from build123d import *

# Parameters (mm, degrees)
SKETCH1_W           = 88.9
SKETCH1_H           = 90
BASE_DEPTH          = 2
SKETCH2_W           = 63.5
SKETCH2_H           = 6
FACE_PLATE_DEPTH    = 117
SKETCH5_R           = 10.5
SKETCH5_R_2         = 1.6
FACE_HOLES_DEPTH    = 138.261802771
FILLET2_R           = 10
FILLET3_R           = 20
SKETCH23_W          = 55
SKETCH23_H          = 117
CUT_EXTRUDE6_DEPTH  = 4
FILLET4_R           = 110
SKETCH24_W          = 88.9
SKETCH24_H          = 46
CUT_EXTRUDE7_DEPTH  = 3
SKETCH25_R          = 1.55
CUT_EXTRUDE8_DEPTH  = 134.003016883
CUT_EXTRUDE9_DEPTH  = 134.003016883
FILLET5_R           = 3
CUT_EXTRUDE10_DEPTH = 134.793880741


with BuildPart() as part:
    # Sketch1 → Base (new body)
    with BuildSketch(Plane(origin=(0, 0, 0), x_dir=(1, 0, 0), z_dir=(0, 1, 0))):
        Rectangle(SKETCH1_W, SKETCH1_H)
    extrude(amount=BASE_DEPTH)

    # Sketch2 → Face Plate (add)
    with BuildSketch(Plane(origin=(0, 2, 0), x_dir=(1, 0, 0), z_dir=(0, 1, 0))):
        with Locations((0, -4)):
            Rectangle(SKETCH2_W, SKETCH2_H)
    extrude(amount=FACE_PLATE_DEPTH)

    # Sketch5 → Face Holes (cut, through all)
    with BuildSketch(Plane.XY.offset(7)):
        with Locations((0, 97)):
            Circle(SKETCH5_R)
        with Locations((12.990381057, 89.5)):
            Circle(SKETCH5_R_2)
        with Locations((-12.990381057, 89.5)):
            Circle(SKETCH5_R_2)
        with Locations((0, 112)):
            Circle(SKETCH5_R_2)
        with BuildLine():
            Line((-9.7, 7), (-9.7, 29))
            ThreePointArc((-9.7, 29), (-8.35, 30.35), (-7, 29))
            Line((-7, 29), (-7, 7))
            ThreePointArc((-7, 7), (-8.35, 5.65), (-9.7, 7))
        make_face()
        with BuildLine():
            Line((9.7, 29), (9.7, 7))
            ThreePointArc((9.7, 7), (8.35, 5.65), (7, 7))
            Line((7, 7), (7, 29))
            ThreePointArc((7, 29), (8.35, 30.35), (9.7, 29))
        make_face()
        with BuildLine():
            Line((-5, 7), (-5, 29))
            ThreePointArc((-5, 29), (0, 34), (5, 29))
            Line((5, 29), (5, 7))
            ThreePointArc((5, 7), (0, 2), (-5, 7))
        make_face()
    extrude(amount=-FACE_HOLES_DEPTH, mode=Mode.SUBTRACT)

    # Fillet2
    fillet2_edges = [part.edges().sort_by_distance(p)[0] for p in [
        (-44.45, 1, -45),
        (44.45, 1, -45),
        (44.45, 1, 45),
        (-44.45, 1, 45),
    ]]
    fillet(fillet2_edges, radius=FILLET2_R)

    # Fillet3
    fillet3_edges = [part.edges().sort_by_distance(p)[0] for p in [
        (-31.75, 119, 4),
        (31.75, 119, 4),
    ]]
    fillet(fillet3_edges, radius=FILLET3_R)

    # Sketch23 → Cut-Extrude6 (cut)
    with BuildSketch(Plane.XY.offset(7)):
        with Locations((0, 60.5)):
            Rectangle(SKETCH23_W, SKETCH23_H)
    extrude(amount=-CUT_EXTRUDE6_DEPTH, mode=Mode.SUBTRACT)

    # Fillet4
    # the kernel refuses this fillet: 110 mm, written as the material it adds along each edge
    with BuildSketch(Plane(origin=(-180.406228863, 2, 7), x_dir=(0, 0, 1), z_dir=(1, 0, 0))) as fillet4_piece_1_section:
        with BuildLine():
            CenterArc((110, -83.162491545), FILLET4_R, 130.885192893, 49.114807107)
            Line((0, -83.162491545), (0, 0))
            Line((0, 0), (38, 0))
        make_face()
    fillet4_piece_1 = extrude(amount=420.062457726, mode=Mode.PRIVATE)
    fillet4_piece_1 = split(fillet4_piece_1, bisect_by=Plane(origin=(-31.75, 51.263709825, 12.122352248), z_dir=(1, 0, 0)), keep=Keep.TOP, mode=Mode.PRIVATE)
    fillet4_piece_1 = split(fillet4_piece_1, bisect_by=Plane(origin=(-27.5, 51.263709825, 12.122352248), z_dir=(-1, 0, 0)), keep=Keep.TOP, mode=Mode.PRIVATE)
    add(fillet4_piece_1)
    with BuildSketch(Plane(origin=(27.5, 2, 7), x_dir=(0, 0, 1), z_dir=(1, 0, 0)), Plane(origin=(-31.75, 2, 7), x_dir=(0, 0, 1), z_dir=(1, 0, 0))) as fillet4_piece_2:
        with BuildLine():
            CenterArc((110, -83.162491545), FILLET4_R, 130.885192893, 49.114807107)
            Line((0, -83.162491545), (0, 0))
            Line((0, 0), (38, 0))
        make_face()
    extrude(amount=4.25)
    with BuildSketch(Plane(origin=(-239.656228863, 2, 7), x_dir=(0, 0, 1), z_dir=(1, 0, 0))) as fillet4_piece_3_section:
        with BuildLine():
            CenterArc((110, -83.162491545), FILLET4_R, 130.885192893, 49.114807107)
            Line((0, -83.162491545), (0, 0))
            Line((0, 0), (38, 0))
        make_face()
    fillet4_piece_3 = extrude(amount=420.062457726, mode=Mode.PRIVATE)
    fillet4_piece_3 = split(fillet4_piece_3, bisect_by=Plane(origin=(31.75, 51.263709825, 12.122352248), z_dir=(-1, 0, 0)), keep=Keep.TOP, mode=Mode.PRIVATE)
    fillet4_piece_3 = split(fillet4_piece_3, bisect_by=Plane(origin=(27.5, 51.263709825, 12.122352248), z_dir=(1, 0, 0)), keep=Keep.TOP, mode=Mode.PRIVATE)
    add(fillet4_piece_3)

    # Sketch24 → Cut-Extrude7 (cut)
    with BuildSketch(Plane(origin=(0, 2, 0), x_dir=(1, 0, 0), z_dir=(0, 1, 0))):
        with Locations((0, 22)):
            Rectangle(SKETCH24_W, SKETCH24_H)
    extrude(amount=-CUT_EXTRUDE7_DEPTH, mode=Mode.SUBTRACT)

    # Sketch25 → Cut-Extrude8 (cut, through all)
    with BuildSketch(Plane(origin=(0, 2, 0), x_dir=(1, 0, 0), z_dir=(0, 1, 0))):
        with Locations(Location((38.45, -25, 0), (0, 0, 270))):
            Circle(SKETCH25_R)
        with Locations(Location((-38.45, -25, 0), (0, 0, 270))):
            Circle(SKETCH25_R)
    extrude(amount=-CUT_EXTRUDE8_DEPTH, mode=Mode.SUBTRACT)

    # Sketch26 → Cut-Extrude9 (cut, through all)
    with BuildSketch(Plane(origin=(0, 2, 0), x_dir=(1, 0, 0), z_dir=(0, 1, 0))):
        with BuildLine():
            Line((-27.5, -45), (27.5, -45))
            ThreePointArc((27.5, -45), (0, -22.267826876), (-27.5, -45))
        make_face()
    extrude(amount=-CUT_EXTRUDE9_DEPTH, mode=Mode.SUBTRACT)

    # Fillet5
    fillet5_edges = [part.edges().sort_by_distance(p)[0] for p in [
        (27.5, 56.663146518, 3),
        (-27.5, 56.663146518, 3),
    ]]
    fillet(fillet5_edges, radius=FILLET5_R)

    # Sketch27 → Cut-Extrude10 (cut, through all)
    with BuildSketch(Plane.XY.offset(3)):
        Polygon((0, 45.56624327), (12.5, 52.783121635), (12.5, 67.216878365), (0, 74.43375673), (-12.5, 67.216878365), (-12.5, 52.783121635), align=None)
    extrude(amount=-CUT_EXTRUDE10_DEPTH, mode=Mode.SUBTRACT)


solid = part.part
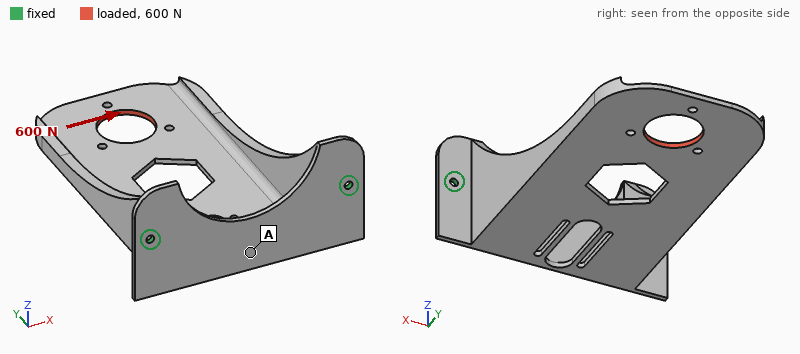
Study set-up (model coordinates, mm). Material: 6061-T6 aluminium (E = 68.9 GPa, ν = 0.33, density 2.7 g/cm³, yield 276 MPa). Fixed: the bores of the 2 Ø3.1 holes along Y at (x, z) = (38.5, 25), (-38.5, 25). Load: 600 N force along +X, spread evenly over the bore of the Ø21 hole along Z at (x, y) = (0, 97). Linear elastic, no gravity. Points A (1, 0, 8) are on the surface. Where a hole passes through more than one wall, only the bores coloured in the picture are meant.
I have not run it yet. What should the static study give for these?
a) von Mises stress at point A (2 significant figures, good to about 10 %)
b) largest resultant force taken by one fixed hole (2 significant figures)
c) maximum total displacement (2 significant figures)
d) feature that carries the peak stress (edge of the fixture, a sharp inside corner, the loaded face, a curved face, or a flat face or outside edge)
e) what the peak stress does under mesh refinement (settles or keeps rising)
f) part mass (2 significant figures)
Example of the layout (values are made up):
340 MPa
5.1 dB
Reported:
51 MPa
850 N
1.7 mm
edge of the fixture
keeps rising
81 g
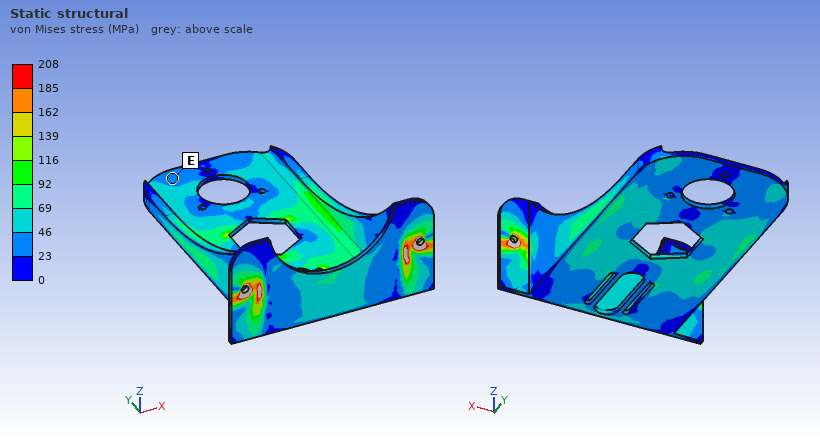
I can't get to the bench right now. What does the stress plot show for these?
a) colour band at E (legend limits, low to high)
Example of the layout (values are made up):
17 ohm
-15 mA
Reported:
23 to 46 MPa
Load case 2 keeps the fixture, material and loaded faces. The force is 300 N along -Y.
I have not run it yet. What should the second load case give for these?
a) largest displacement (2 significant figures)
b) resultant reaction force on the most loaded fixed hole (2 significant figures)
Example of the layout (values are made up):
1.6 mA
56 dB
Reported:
1.3 mm
150 N
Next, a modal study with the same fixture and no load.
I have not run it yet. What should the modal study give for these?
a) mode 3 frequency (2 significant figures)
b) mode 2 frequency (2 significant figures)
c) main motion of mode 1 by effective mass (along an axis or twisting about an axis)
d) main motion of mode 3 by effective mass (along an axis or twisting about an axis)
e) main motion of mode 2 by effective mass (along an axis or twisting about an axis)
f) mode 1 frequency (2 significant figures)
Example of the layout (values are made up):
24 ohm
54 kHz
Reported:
1700 Hz
560 Hz
along Z
along Y
along X
260 Hz
